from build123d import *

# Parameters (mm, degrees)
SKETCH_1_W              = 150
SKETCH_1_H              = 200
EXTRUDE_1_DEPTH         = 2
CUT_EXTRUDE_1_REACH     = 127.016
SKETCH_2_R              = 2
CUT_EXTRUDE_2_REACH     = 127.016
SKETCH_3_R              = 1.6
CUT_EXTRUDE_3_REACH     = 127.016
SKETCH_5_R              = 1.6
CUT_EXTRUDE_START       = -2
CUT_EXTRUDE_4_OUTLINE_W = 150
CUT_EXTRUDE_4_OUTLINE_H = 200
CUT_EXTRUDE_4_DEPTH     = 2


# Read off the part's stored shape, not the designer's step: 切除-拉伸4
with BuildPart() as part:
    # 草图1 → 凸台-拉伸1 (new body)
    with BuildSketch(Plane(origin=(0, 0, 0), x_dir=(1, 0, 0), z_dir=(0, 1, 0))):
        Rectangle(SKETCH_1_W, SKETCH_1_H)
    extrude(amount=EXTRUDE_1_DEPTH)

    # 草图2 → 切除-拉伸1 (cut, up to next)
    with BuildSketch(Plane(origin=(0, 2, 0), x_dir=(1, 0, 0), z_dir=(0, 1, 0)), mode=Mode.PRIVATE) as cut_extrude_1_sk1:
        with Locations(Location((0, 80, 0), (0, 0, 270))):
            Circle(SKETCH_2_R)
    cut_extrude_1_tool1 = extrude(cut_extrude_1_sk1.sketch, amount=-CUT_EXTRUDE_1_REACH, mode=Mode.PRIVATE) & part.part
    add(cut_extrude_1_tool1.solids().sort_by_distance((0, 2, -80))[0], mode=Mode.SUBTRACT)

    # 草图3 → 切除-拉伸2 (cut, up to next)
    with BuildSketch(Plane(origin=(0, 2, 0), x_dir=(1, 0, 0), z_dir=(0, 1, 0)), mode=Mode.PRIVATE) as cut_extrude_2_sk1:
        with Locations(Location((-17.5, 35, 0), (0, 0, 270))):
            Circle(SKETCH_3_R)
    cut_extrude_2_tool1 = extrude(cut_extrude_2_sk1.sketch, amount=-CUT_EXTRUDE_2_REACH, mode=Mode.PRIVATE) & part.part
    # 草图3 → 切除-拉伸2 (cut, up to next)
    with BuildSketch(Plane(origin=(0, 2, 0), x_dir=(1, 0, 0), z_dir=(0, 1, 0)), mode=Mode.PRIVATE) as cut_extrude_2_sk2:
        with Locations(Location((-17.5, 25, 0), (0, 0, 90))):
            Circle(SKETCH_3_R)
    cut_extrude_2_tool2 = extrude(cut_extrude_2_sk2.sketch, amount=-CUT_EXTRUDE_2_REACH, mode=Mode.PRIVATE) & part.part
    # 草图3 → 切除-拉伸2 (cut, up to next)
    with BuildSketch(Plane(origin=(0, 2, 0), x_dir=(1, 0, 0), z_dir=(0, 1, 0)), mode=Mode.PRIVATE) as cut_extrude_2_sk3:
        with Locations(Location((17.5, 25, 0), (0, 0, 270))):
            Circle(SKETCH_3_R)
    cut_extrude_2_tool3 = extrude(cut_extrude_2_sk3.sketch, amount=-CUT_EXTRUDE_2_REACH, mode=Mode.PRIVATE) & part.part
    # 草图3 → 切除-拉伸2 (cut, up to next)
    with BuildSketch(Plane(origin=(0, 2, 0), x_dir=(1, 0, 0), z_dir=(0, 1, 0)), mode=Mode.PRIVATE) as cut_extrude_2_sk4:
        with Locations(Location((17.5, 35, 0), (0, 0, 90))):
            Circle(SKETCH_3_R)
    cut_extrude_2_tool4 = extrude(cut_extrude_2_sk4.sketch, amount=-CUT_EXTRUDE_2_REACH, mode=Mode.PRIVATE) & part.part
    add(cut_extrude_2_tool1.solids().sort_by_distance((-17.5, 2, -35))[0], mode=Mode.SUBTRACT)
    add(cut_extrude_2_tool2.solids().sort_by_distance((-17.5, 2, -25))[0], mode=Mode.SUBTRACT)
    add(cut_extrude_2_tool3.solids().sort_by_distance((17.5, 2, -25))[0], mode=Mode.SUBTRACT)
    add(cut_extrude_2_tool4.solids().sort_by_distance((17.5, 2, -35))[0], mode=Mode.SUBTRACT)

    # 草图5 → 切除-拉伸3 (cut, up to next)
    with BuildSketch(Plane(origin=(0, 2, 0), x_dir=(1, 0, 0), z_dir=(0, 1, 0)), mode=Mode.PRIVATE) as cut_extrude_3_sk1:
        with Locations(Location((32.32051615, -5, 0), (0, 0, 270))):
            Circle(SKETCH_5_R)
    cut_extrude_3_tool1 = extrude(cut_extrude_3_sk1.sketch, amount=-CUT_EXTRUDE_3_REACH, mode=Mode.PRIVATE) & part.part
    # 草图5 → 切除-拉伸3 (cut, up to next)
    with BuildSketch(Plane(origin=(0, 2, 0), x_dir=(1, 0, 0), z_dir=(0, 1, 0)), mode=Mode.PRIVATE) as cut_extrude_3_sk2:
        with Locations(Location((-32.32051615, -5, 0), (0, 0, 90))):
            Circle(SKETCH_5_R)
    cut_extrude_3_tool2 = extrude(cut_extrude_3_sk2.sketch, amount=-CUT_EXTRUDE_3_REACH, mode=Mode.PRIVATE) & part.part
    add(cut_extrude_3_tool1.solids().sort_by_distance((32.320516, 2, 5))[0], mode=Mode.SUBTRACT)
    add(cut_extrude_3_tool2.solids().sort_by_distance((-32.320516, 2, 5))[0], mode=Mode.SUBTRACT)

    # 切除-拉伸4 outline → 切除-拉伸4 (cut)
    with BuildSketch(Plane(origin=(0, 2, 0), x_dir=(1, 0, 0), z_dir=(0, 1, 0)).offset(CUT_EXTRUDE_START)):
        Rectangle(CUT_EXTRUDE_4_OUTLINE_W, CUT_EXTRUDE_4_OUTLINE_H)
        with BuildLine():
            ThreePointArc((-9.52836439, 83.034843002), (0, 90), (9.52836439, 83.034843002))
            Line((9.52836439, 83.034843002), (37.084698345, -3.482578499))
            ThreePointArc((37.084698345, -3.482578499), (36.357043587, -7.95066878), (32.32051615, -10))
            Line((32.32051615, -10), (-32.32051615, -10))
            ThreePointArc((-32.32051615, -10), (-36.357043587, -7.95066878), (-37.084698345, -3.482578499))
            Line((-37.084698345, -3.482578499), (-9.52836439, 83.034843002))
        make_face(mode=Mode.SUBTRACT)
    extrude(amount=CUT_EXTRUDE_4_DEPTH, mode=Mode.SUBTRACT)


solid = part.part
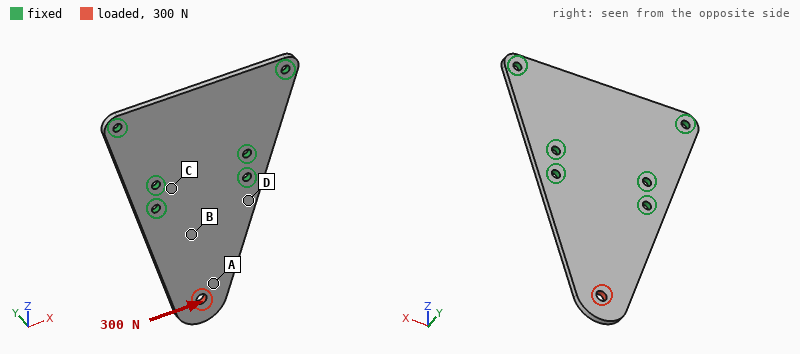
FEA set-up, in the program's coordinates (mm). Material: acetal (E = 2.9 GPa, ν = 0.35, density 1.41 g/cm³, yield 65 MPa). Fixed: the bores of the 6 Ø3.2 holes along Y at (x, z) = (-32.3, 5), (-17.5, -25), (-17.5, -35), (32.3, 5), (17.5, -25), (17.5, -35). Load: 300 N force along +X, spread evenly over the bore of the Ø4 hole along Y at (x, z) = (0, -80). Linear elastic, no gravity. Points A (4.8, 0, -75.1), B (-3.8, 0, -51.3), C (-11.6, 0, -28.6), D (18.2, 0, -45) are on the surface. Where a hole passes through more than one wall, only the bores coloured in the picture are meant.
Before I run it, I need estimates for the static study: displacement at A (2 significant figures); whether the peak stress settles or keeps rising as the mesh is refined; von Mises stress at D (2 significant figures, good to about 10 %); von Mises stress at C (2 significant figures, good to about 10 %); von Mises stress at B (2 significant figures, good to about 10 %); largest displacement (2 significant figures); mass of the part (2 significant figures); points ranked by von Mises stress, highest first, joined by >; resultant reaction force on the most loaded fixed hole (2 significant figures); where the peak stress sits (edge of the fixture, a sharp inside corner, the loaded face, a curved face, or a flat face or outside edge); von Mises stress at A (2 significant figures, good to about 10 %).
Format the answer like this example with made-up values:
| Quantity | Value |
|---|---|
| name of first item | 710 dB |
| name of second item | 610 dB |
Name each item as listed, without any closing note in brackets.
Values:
| Quantity | Value |
|---|---|
| displacement at A | 0.40 mm |
| whether the peak stress settles or keeps rising as the mesh is refined | keeps rising |
| von Mises stress at D | 16 MPa |
| von Mises stress at C | 2.7 MPa |
| von Mises stress at B | 6.5 MPa |
| largest displacement | 0.61 mm |
| mass of the part | 13 g |
| points ranked by von Mises stress, highest first, joined by > | D > A > B > C |
| resultant reaction force on the most loaded fixed hole | 320 N |
| where the peak stress sits | edge of the fixture |
| von Mises stress at A | 12 MPa |
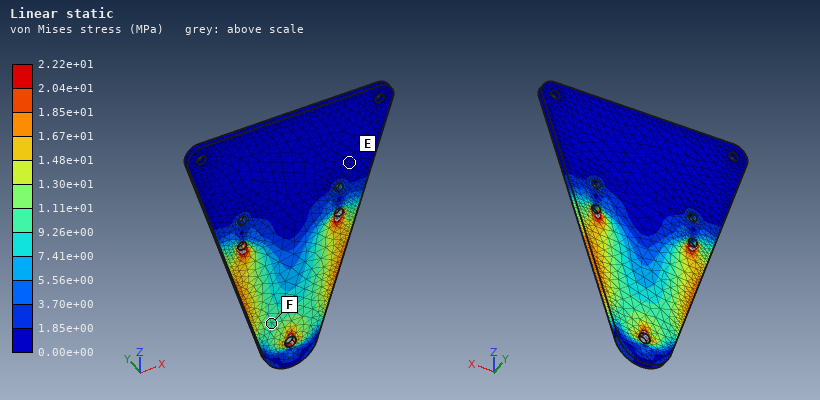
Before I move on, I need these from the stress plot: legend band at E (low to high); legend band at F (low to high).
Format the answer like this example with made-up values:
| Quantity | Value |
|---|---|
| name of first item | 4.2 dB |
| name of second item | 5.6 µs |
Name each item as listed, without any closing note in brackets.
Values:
| Quantity | Value |
|---|---|
| legend band at E | 0.00e+00 to 1.85e+00 MPa |
| legend band at F | 9.26e+00 to 1.11e+01 MPa |
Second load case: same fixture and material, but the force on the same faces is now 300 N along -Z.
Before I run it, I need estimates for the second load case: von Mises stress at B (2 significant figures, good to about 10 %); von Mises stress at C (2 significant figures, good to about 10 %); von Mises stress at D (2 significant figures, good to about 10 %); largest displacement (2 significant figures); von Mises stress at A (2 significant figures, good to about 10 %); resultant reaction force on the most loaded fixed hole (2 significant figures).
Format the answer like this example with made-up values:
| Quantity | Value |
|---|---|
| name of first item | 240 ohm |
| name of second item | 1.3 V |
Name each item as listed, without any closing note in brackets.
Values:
| Quantity | Value |
|---|---|
| von Mises stress at B | 3.8 MPa |
| von Mises stress at C | 2.3 MPa |
| von Mises stress at D | 4.1 MPa |
| largest displacement | 0.11 mm |
| von Mises stress at A | 7.6 MPa |
| resultant reaction force on the most loaded fixed hole | 100 N |
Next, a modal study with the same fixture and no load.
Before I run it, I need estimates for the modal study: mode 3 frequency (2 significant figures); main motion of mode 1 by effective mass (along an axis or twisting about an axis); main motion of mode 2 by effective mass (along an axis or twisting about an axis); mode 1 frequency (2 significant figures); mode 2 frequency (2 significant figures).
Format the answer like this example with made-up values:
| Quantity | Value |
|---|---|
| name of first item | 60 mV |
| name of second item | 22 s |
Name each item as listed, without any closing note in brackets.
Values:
| Quantity | Value |
|---|---|
| mode 3 frequency | 940 Hz |
| main motion of mode 1 by effective mass | along Y |
| main motion of mode 2 by effective mass | along Y |
| mode 1 frequency | 220 Hz |
| mode 2 frequency | 890 Hz |
